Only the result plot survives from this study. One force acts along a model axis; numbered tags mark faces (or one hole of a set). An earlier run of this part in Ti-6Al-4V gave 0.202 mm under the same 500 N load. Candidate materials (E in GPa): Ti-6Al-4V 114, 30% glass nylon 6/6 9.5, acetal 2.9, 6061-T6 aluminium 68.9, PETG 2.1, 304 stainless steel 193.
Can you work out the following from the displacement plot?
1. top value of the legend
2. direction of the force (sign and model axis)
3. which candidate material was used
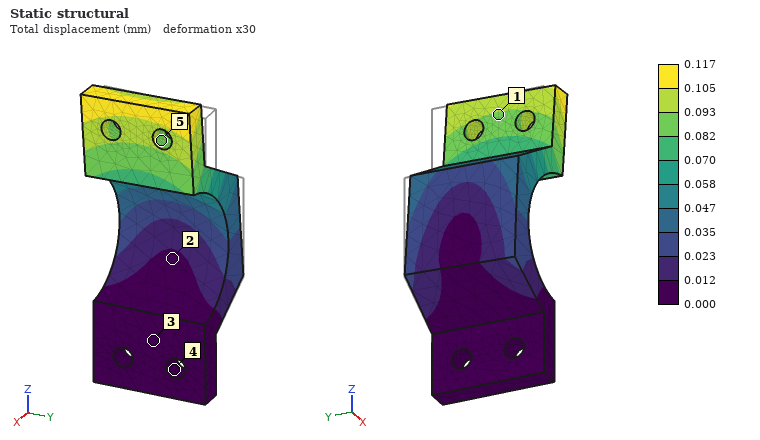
0.117 mm
-Y
304 stainless steel
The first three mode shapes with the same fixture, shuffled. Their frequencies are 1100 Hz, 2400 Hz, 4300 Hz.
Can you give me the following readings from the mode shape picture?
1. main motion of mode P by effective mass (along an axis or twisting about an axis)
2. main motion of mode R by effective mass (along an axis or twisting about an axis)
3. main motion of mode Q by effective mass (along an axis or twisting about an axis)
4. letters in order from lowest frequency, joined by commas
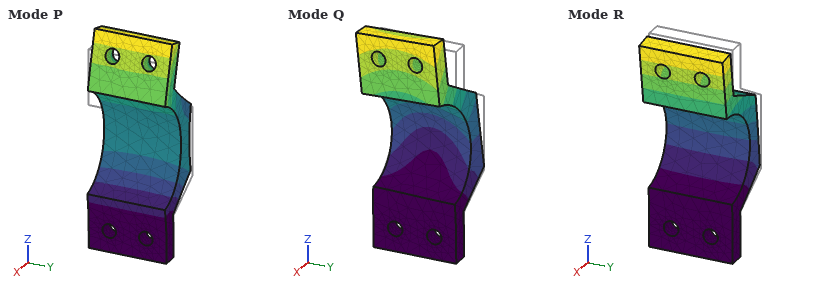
along Z
along X
along Y
R, Q, P
